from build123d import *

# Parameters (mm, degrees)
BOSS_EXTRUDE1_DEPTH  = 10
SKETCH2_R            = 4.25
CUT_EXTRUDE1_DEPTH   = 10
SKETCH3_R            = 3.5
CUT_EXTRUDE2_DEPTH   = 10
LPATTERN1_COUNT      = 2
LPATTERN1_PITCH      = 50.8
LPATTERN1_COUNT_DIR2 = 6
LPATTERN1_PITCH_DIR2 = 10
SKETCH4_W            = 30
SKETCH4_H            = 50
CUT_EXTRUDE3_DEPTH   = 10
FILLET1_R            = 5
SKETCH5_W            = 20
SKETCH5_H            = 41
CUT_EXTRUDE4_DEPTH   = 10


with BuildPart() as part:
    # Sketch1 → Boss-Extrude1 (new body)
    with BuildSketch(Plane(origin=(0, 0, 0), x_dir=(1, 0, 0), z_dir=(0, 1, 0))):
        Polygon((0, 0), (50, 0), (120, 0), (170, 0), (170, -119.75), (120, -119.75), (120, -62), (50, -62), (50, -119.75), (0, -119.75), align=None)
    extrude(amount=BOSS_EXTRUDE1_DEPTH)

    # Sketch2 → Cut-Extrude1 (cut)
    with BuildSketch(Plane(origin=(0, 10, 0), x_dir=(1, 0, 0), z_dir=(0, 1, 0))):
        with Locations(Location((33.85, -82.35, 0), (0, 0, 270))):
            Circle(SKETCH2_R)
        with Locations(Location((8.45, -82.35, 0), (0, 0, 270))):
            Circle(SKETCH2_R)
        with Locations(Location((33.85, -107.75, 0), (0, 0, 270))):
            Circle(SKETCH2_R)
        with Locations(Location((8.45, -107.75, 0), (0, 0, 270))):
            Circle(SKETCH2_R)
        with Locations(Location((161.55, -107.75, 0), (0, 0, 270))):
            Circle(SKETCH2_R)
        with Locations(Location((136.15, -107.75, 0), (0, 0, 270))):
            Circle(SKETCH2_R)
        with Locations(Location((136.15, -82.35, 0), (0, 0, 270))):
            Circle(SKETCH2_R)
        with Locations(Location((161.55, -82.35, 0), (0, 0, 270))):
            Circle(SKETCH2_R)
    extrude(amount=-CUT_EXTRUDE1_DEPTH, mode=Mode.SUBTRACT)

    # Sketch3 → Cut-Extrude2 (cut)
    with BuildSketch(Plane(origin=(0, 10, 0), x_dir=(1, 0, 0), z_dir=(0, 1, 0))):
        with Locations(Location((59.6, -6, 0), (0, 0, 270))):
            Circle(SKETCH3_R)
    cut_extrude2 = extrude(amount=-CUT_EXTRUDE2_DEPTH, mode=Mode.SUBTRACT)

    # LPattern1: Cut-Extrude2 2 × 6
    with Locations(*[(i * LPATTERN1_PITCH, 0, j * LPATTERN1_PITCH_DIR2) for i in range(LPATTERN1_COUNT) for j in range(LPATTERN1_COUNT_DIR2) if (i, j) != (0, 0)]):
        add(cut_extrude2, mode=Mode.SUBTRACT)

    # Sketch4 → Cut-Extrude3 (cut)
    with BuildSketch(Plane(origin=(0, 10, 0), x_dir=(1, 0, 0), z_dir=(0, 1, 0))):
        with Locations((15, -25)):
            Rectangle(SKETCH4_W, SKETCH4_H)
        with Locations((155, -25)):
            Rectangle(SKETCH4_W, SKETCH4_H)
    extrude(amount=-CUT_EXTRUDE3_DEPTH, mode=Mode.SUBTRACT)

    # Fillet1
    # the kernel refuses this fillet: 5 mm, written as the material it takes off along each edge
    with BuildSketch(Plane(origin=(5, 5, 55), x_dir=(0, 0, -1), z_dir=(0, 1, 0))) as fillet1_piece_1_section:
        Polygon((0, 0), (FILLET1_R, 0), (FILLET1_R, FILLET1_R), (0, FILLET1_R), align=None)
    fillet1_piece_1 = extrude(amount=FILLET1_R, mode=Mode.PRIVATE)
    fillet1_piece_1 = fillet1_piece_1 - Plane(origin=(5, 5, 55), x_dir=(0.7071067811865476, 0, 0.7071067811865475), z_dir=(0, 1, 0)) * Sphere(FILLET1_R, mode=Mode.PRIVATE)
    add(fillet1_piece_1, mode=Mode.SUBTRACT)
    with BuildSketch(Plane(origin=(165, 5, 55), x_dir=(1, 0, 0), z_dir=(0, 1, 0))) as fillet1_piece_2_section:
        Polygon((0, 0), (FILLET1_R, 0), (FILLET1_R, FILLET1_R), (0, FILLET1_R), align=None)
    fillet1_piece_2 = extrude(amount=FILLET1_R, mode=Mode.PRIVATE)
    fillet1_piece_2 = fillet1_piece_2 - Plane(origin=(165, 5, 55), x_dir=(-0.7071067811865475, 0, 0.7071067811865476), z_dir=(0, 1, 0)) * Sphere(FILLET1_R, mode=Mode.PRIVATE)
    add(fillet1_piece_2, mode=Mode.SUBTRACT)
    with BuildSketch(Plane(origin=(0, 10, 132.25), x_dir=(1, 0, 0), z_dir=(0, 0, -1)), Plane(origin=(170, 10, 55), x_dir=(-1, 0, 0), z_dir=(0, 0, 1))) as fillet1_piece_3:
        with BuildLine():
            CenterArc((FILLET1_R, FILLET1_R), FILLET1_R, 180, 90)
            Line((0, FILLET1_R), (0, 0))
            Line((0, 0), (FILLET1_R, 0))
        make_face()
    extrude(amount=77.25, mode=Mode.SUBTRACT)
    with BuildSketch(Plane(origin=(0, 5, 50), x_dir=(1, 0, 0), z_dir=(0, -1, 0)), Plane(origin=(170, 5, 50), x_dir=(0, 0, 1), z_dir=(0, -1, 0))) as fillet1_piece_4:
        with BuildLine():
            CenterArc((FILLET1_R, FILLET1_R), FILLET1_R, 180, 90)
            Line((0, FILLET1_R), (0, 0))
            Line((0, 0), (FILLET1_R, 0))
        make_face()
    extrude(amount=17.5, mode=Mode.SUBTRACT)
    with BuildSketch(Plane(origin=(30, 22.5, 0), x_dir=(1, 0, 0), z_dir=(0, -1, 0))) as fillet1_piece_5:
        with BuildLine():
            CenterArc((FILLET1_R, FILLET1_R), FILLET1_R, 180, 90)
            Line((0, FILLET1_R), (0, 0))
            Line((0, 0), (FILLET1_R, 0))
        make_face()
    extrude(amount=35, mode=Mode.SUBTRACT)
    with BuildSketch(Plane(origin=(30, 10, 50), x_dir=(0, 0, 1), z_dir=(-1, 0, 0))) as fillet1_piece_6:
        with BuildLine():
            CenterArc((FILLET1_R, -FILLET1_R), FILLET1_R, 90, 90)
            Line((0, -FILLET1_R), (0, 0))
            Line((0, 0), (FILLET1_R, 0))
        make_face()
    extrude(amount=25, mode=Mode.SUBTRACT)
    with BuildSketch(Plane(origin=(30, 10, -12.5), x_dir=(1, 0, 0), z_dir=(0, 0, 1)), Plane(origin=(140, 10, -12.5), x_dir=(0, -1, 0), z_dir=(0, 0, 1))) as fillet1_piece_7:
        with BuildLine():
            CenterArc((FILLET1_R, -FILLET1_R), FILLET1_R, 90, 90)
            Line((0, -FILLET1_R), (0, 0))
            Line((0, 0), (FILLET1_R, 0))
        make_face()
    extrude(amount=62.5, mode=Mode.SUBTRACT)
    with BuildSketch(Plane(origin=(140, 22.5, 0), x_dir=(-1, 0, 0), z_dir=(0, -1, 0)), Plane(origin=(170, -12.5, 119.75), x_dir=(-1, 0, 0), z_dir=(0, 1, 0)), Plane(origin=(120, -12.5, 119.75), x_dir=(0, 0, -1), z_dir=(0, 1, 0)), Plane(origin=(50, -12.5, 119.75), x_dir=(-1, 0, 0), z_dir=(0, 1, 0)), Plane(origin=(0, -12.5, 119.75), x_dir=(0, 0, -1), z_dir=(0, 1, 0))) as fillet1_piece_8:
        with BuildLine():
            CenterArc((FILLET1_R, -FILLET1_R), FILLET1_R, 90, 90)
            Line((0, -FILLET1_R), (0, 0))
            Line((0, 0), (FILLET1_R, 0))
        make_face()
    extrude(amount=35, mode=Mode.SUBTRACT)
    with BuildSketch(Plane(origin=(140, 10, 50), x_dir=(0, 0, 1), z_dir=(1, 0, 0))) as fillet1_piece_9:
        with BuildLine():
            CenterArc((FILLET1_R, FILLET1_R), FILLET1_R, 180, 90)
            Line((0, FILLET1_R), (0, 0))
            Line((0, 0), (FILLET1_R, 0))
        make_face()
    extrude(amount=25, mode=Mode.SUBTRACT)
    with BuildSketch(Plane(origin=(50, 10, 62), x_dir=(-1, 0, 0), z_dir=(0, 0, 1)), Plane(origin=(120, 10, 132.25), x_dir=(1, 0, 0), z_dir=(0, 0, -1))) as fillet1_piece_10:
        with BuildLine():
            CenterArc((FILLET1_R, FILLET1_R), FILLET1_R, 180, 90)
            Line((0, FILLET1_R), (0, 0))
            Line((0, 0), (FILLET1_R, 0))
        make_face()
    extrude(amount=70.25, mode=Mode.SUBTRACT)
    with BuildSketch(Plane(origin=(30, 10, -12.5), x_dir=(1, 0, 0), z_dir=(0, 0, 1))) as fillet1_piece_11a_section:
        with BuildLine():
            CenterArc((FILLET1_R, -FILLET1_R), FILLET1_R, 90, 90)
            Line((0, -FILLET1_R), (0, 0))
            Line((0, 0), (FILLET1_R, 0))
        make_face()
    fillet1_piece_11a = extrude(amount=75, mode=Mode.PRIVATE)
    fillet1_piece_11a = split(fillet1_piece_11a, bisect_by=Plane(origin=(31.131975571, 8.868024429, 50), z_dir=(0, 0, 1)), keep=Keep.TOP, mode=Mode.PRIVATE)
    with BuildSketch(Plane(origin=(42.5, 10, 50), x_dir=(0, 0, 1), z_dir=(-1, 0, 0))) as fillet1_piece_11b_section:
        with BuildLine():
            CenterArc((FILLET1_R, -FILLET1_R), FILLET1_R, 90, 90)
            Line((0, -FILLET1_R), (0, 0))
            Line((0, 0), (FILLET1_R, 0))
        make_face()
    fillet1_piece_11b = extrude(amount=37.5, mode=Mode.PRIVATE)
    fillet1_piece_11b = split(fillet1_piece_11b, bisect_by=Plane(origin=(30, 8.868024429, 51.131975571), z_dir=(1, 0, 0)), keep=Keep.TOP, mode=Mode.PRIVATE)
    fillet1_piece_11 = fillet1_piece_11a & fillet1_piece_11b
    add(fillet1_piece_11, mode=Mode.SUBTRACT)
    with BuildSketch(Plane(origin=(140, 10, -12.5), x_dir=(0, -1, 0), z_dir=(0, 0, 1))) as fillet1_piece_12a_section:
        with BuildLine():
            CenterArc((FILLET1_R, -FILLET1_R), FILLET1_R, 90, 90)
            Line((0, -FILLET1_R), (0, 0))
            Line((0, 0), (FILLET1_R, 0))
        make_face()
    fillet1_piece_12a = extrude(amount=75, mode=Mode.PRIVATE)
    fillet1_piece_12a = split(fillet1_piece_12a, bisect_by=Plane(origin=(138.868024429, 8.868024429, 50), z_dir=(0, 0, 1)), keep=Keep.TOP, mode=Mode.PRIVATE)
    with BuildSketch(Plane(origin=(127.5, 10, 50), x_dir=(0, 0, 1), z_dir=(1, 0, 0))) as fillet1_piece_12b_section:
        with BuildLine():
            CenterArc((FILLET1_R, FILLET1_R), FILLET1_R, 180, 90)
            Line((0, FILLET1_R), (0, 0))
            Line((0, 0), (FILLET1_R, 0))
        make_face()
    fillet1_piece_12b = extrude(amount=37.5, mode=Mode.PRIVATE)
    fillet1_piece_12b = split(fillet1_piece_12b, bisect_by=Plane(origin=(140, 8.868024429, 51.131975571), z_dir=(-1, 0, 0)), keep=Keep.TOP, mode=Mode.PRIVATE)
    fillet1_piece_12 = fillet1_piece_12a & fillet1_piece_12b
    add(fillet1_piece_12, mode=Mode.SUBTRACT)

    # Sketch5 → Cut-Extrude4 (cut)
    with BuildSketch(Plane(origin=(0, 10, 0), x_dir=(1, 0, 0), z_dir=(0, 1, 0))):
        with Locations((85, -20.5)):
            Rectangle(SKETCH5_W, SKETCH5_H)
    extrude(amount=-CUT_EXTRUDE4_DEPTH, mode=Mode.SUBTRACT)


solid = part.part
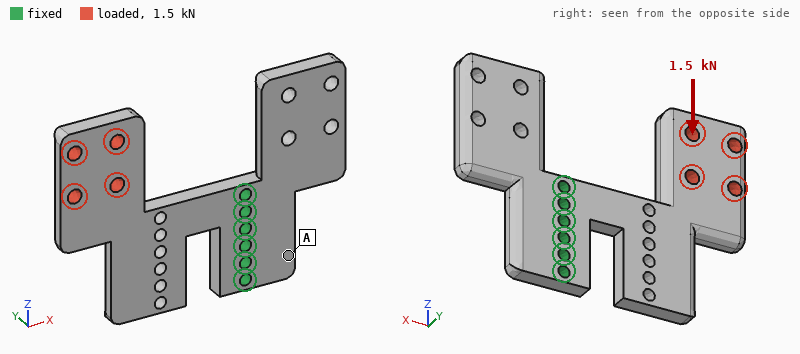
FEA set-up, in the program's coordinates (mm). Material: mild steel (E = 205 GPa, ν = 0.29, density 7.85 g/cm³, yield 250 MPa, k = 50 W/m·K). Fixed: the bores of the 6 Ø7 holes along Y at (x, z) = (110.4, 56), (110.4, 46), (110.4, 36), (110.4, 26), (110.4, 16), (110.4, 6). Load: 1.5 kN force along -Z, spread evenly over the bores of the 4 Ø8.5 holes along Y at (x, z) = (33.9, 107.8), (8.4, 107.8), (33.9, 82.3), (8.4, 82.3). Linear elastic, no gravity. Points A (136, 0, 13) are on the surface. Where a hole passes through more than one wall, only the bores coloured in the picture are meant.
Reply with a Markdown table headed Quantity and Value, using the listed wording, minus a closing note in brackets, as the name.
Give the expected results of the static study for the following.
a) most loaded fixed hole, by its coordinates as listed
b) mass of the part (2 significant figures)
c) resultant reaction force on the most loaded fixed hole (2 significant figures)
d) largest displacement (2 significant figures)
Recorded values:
| Quantity | Value |
|---|---|
| most loaded fixed hole, by its coordinates as listed | (110.4, 56) |
| mass of the part | 890 g |
| resultant reaction force on the most loaded fixed hole | 6.6 kN |
| largest displacement | 0.30 mm |
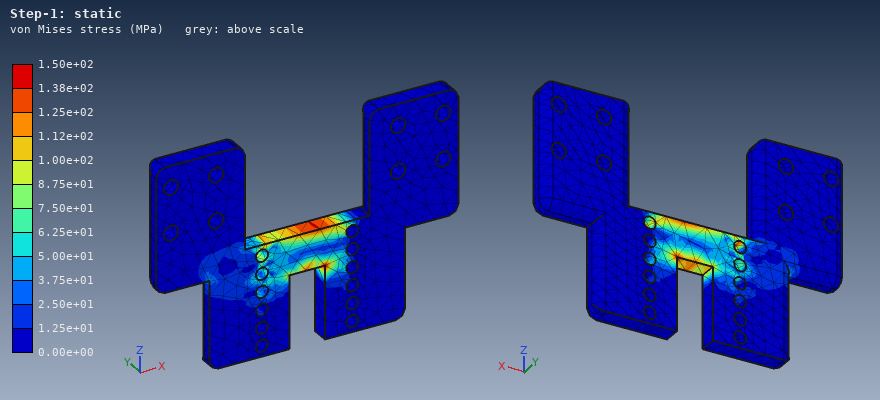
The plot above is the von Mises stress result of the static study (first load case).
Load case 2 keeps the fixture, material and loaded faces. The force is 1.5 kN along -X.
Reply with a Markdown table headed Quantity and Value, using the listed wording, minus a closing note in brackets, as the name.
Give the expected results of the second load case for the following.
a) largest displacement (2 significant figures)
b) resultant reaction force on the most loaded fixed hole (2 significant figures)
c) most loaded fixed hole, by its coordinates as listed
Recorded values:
| Quantity | Value |
|---|---|
| largest displacement | 0.24 mm |
| resultant reaction force on the most loaded fixed hole | 4.3 kN |
| most loaded fixed hole, by its coordinates as listed | (110.4, 56) |
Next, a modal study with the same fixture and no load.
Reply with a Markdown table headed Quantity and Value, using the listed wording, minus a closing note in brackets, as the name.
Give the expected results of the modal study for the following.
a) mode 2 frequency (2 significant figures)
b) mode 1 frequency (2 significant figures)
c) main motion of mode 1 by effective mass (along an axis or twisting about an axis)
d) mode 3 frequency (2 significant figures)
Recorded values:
| Quantity | Value |
|---|---|
| mode 2 frequency | 730 Hz |
| mode 1 frequency | 370 Hz |
| main motion of mode 1 by effective mass | along Y |
| mode 3 frequency | 760 Hz |
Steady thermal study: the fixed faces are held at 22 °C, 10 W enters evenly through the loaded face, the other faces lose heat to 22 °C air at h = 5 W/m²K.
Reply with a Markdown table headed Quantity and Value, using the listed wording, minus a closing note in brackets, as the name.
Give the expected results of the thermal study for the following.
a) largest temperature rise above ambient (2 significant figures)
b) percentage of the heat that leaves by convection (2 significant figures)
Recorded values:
| Quantity | Value |
|---|---|
| largest temperature rise above ambient | 61 K |
| percentage of the heat that leaves by convection | 34 % |
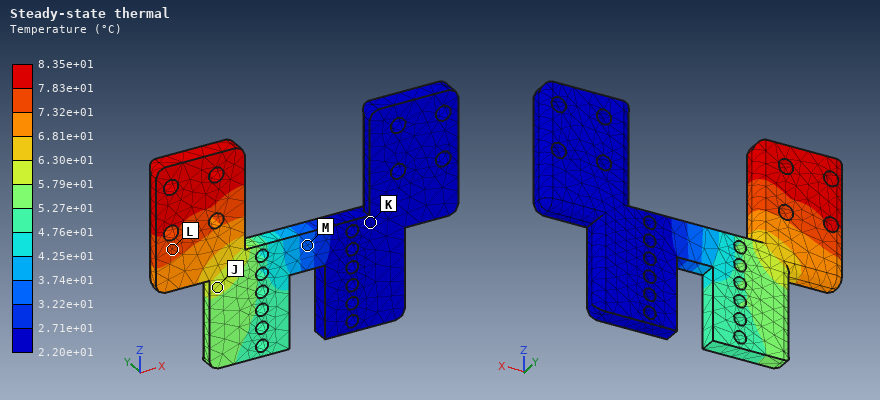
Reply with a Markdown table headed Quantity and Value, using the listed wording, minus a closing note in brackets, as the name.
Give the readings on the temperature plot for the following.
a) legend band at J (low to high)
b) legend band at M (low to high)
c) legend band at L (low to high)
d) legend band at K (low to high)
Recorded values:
| Quantity | Value |
|---|---|
| legend band at J | 5.79e+01 to 6.30e+01 °C |
| legend band at M | 3.22e+01 to 3.74e+01 °C |
| legend band at L | 7.32e+01 to 7.83e+01 °C |
| legend band at K | 2.20e+01 to 2.71e+01 °C |
